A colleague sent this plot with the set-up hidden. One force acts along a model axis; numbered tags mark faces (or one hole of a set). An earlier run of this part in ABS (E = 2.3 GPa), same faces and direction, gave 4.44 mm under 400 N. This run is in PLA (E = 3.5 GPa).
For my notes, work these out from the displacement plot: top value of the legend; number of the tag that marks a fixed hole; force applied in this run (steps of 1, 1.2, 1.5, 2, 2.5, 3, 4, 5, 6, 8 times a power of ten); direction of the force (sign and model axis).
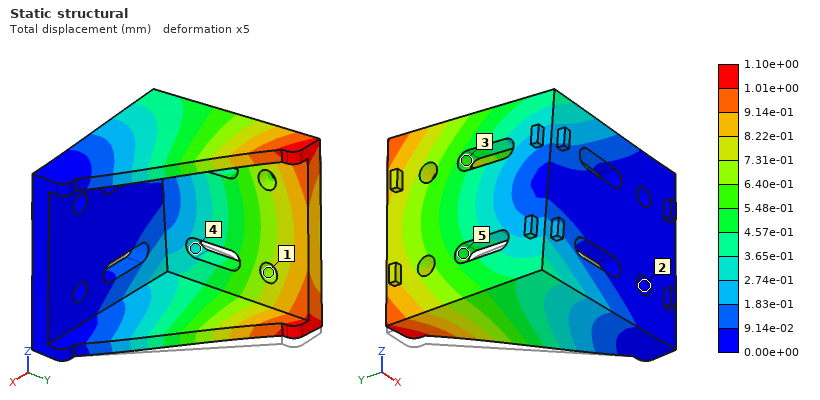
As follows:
1.10e+00 mm
2
150 N
+Z
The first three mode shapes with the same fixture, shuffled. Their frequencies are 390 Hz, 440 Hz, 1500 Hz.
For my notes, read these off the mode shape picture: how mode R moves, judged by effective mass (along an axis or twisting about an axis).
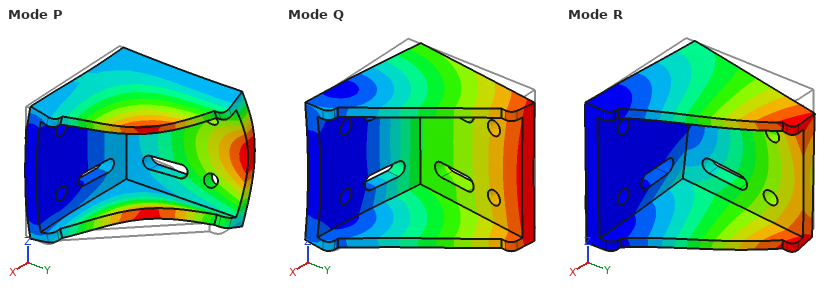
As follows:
along Z
